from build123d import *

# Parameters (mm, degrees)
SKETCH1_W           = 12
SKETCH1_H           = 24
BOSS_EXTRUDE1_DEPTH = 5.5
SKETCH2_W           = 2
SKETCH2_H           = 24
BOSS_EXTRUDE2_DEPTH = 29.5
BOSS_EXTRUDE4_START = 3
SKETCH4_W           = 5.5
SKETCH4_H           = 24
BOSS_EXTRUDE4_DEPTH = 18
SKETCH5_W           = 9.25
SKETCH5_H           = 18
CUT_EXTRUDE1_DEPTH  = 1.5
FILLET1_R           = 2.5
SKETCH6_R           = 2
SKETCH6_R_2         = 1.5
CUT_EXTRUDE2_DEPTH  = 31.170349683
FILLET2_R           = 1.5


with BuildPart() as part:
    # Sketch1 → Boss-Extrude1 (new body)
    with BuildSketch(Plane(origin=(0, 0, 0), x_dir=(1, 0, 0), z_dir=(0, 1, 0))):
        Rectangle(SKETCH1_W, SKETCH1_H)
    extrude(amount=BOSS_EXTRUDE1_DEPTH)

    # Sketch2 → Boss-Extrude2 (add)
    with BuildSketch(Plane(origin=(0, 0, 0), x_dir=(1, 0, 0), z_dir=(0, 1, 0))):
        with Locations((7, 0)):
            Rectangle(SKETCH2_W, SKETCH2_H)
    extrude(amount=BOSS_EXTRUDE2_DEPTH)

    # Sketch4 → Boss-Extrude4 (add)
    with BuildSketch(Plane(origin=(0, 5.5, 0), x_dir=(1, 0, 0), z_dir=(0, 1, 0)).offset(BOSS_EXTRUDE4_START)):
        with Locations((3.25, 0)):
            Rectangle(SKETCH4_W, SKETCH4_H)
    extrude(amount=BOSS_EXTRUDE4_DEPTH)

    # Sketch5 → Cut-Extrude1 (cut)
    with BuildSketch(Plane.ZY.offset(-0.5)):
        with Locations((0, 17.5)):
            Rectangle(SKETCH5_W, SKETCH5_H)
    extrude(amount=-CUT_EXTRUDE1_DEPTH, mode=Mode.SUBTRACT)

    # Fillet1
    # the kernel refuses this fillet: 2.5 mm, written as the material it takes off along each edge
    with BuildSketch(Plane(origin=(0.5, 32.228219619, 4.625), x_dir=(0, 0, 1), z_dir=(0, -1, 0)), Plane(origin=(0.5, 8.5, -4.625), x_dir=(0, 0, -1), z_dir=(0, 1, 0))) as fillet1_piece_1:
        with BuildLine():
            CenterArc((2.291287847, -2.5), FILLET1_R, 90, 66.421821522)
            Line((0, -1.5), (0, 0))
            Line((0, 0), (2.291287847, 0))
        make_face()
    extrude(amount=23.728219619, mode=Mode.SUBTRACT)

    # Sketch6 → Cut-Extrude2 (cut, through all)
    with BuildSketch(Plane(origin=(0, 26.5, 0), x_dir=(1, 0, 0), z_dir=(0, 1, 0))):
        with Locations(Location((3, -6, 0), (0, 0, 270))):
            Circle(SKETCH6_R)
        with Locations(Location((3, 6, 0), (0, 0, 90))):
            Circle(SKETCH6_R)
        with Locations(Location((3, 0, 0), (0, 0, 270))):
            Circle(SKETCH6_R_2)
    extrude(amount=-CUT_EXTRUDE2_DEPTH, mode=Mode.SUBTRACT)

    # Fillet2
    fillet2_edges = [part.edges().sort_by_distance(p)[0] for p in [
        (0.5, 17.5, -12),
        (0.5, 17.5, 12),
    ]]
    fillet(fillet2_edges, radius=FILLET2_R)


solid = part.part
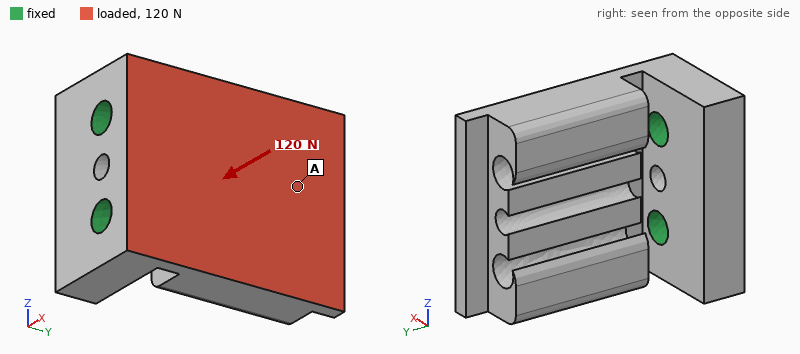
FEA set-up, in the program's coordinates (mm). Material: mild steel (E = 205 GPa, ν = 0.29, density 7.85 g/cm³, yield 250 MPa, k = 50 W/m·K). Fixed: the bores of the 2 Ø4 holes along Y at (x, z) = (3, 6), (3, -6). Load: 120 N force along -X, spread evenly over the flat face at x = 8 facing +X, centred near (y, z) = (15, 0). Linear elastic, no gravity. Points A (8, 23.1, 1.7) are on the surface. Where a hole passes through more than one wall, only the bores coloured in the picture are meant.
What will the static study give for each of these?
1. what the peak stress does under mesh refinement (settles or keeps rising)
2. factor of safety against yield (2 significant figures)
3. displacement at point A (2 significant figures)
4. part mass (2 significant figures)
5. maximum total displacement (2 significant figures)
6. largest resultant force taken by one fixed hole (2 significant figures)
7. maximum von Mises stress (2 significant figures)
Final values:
settles
3.9
26 µm
34 g
37 µm
60 N
64 MPa
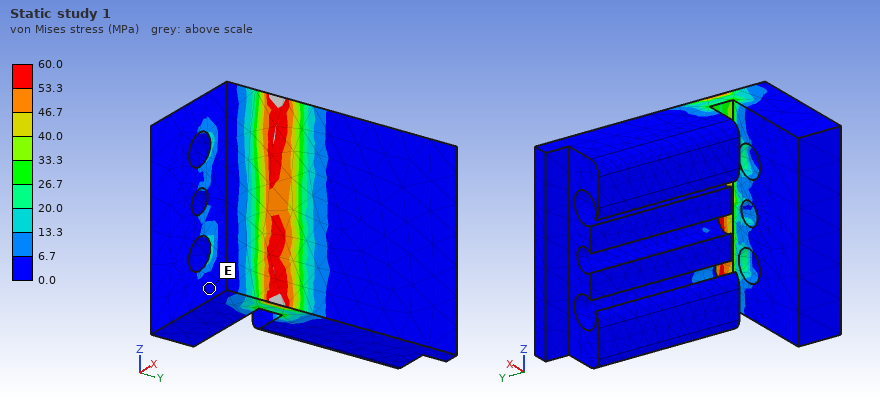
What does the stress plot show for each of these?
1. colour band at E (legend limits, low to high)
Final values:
0.0 to 6.7 MPa
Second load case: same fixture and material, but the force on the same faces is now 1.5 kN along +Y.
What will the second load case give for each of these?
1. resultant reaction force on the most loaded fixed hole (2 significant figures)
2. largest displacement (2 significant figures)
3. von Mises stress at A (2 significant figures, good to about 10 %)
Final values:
750 N
53 µm
12 MPa
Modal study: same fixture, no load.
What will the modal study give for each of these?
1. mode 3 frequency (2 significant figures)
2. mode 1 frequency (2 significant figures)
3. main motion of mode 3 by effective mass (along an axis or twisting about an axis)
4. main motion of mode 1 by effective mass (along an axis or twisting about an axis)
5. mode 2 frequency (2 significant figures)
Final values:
12 kHz
2300 Hz
along Z
along X
8100 Hz
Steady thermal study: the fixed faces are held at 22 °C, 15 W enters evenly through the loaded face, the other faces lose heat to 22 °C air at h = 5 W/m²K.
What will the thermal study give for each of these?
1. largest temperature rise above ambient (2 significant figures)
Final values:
49 K
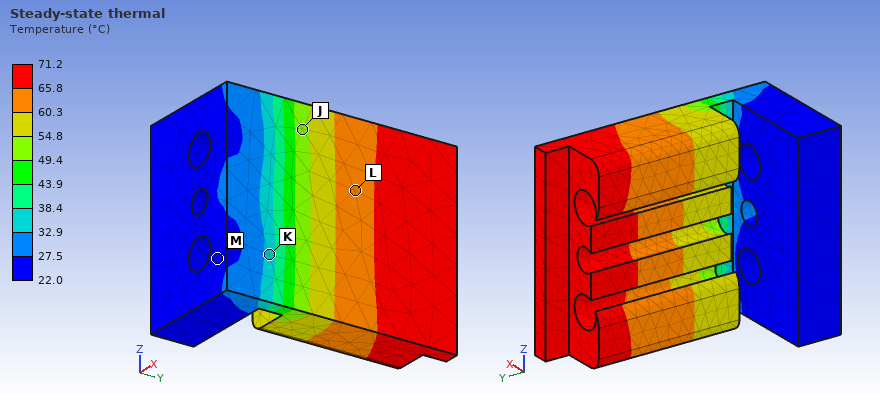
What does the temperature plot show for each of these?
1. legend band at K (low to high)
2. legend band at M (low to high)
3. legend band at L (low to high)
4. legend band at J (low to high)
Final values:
32.9 to 38.4 °C
22.0 to 27.5 °C
60.3 to 65.8 °C
49.4 to 54.8 °C
